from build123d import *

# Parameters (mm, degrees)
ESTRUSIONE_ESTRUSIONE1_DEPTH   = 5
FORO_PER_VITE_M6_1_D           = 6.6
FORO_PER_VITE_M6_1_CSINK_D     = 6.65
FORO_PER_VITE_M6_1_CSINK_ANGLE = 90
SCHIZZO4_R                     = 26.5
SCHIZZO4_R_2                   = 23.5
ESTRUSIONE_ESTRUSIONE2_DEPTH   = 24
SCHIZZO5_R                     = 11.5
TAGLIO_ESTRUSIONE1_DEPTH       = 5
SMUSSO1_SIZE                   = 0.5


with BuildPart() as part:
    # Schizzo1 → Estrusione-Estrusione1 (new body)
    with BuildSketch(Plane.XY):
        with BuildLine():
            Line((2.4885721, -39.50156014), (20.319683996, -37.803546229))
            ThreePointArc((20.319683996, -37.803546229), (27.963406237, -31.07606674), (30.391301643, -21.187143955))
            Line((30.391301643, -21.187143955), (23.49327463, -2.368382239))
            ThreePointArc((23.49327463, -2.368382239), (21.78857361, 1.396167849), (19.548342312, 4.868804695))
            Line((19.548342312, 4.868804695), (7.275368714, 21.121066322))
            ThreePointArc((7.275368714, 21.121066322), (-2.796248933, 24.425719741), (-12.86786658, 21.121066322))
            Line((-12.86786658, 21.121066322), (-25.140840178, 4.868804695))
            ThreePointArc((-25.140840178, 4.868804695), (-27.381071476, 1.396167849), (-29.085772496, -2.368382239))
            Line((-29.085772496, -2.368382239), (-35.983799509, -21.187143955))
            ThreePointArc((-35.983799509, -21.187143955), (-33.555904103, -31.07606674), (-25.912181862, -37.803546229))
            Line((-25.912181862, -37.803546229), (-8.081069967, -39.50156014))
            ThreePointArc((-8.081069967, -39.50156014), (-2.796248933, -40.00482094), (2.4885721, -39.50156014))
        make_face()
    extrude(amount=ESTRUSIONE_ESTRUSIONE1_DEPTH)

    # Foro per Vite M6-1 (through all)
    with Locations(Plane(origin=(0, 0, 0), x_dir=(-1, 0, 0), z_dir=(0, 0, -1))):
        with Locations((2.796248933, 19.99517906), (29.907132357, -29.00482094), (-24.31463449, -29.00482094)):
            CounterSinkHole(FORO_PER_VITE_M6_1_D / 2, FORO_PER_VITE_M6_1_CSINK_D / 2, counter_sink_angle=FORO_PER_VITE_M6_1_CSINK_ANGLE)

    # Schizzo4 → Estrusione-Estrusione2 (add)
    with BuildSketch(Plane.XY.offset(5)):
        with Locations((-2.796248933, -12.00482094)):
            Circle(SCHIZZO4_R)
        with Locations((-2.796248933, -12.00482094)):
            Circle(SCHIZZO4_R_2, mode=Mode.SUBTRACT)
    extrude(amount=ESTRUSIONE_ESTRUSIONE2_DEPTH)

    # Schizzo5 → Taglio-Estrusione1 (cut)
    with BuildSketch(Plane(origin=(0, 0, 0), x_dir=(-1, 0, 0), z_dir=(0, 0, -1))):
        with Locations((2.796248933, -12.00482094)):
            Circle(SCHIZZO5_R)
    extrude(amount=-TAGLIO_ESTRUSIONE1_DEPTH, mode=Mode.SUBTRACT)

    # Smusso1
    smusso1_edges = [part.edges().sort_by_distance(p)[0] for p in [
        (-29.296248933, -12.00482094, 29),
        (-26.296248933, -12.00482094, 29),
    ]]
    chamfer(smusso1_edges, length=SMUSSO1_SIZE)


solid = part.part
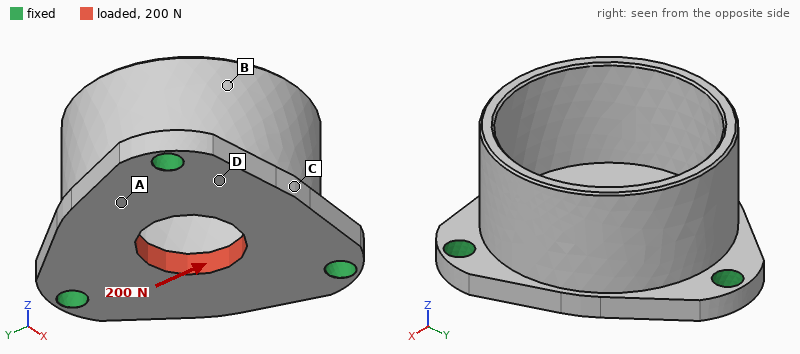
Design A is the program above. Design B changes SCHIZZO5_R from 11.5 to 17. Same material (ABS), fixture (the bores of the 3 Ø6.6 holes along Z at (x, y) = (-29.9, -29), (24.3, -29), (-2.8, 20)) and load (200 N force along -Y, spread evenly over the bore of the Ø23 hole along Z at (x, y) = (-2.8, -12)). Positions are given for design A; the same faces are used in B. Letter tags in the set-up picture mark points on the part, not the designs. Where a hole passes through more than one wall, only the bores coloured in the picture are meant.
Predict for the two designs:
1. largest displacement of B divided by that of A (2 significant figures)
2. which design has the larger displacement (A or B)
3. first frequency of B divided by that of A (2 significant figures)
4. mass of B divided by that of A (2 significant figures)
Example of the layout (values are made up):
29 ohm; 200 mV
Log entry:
1.3; B; 0.99; 0.90
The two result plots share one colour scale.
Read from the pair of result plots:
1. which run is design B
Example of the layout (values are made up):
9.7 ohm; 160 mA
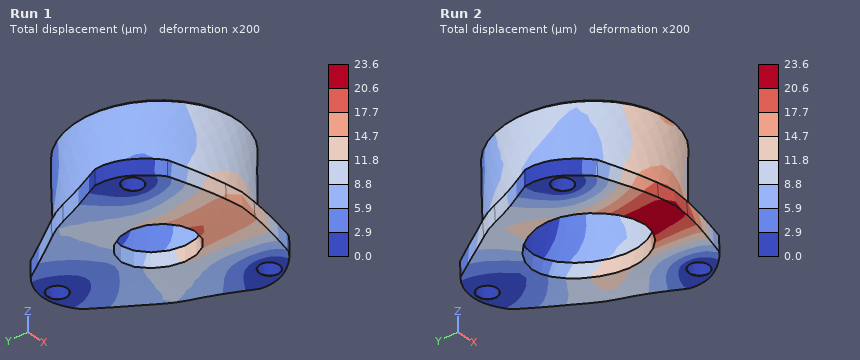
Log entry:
Run 2
